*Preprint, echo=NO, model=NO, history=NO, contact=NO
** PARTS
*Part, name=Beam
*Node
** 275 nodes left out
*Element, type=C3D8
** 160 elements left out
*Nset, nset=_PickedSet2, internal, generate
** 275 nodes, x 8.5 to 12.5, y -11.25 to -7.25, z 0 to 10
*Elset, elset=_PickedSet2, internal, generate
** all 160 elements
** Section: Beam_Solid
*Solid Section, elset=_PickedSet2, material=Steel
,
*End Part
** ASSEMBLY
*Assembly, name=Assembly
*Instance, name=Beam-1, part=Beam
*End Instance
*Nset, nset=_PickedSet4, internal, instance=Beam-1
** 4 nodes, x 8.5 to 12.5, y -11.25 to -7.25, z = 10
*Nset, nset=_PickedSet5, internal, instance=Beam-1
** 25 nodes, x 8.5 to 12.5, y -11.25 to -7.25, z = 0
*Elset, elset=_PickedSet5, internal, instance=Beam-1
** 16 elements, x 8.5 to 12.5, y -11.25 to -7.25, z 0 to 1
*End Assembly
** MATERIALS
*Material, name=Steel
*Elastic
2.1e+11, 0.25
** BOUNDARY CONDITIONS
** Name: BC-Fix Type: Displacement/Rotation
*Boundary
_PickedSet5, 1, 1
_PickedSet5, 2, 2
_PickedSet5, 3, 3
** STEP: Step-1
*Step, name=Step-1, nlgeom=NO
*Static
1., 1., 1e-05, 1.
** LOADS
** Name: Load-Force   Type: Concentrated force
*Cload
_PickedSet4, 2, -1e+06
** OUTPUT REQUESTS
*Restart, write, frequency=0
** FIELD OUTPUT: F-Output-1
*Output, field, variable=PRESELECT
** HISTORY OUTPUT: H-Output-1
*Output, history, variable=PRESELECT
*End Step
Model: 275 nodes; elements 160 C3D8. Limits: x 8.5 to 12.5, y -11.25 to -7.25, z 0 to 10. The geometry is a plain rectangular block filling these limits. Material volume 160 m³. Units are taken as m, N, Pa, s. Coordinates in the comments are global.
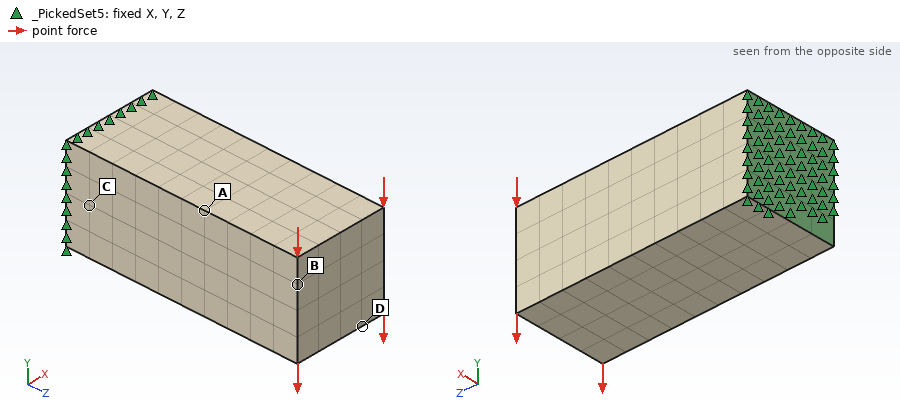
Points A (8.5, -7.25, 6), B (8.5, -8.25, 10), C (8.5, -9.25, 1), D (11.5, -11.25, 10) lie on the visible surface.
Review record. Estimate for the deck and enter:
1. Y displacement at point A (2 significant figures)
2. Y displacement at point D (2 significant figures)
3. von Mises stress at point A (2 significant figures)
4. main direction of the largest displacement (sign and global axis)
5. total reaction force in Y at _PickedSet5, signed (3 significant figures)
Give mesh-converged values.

-1.5e-04 m
-3.3e-04 m
1.5e+06 Pa
-Y
4.00e+06 N
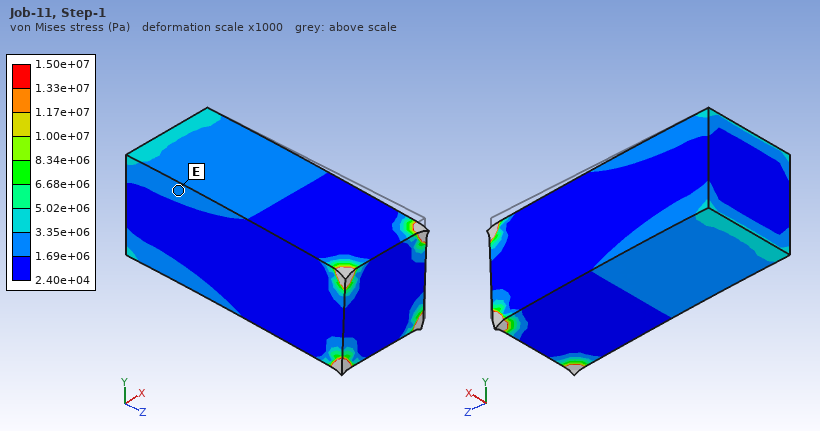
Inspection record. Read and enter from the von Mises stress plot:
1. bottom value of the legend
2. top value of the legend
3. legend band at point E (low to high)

2.40e+04 Pa
1.50e+07 Pa
1.69e+06 to 3.35e+06 Pa
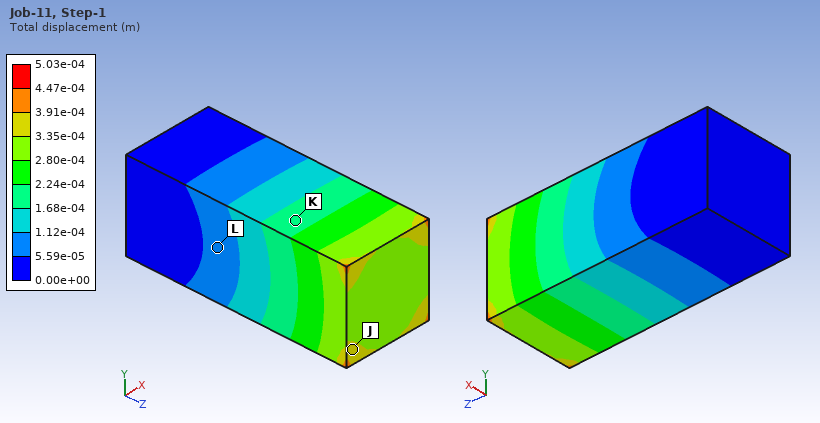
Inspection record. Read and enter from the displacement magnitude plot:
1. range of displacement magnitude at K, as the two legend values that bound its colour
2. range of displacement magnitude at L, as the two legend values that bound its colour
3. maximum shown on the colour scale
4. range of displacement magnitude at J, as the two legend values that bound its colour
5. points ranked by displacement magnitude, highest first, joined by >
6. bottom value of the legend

1.68e-04 to 2.24e-04 m
5.59e-05 to 1.12e-04 m
5.03e-04 m
3.35e-04 to 3.91e-04 m
J > K > L
0.00e+00 m
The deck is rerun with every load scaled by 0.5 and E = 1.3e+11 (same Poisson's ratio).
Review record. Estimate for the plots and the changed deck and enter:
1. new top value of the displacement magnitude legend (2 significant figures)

4.1e-04 m
